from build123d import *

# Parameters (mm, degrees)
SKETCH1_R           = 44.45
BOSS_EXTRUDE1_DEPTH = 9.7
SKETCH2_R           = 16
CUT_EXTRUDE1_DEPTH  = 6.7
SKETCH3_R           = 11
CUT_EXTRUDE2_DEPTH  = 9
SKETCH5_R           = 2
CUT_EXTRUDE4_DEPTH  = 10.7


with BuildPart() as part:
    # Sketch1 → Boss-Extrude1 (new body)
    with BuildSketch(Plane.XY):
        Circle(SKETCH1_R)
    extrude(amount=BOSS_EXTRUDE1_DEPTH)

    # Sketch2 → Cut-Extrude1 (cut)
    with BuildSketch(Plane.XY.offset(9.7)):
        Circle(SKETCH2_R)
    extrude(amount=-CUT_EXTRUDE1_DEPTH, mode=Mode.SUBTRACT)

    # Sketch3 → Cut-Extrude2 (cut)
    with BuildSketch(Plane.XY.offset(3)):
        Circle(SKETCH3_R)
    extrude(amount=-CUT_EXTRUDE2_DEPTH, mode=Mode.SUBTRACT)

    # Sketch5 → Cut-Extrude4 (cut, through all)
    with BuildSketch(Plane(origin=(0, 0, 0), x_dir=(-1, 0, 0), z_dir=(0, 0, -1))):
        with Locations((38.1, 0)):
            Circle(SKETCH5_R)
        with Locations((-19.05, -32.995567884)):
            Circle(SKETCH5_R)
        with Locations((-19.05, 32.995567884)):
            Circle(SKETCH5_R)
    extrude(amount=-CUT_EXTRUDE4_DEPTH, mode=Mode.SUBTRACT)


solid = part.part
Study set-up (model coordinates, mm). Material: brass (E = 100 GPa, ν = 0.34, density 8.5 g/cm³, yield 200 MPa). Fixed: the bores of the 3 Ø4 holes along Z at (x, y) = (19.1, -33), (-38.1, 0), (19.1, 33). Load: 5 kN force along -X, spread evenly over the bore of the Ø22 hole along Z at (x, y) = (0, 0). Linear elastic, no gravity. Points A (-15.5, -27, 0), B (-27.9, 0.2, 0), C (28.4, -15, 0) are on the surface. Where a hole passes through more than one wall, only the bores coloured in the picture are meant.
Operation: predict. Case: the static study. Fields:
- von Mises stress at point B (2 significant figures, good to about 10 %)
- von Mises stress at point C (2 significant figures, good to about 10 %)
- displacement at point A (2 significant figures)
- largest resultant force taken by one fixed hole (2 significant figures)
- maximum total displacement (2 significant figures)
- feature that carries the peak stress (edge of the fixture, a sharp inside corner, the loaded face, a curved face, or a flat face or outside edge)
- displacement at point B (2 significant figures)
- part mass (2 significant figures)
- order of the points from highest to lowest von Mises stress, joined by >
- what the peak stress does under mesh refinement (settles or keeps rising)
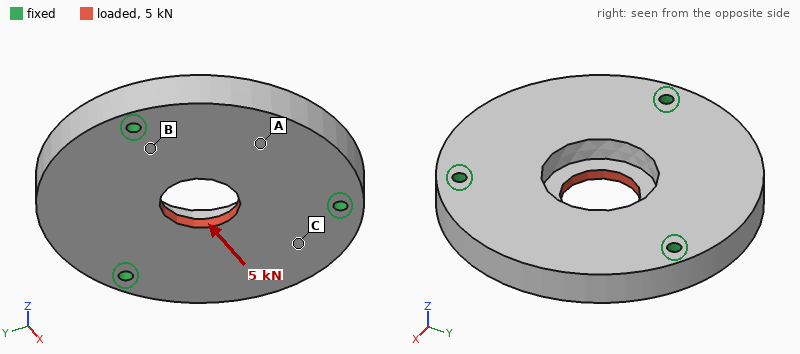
17 MPa
7.1 MPa
2.8 µm
1.7 kN
8.2 µm
edge of the fixture
1.4 µm
450 g
B > C > A
keeps rising
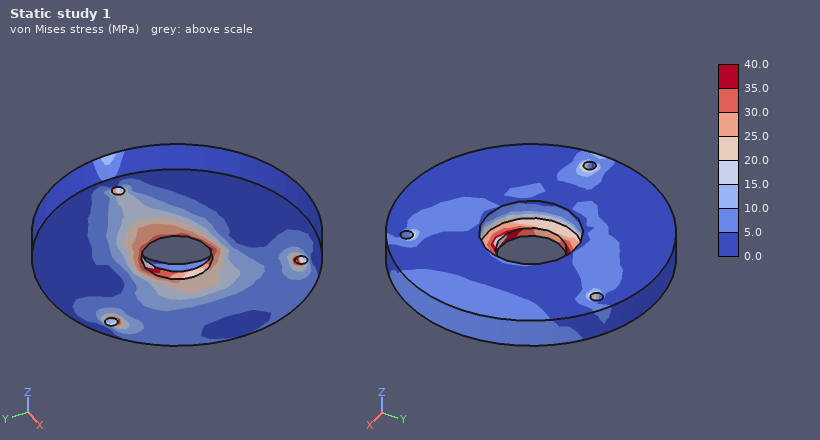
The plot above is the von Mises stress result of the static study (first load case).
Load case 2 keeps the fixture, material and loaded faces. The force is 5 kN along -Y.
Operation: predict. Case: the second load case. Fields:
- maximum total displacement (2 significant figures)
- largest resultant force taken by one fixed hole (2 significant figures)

7.4 µm
1.7 kN
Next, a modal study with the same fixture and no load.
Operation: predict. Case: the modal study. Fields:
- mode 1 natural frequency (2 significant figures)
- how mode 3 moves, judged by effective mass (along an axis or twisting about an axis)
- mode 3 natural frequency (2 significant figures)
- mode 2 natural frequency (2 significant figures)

4400 Hz
along Z
5200 Hz
4400 Hz
